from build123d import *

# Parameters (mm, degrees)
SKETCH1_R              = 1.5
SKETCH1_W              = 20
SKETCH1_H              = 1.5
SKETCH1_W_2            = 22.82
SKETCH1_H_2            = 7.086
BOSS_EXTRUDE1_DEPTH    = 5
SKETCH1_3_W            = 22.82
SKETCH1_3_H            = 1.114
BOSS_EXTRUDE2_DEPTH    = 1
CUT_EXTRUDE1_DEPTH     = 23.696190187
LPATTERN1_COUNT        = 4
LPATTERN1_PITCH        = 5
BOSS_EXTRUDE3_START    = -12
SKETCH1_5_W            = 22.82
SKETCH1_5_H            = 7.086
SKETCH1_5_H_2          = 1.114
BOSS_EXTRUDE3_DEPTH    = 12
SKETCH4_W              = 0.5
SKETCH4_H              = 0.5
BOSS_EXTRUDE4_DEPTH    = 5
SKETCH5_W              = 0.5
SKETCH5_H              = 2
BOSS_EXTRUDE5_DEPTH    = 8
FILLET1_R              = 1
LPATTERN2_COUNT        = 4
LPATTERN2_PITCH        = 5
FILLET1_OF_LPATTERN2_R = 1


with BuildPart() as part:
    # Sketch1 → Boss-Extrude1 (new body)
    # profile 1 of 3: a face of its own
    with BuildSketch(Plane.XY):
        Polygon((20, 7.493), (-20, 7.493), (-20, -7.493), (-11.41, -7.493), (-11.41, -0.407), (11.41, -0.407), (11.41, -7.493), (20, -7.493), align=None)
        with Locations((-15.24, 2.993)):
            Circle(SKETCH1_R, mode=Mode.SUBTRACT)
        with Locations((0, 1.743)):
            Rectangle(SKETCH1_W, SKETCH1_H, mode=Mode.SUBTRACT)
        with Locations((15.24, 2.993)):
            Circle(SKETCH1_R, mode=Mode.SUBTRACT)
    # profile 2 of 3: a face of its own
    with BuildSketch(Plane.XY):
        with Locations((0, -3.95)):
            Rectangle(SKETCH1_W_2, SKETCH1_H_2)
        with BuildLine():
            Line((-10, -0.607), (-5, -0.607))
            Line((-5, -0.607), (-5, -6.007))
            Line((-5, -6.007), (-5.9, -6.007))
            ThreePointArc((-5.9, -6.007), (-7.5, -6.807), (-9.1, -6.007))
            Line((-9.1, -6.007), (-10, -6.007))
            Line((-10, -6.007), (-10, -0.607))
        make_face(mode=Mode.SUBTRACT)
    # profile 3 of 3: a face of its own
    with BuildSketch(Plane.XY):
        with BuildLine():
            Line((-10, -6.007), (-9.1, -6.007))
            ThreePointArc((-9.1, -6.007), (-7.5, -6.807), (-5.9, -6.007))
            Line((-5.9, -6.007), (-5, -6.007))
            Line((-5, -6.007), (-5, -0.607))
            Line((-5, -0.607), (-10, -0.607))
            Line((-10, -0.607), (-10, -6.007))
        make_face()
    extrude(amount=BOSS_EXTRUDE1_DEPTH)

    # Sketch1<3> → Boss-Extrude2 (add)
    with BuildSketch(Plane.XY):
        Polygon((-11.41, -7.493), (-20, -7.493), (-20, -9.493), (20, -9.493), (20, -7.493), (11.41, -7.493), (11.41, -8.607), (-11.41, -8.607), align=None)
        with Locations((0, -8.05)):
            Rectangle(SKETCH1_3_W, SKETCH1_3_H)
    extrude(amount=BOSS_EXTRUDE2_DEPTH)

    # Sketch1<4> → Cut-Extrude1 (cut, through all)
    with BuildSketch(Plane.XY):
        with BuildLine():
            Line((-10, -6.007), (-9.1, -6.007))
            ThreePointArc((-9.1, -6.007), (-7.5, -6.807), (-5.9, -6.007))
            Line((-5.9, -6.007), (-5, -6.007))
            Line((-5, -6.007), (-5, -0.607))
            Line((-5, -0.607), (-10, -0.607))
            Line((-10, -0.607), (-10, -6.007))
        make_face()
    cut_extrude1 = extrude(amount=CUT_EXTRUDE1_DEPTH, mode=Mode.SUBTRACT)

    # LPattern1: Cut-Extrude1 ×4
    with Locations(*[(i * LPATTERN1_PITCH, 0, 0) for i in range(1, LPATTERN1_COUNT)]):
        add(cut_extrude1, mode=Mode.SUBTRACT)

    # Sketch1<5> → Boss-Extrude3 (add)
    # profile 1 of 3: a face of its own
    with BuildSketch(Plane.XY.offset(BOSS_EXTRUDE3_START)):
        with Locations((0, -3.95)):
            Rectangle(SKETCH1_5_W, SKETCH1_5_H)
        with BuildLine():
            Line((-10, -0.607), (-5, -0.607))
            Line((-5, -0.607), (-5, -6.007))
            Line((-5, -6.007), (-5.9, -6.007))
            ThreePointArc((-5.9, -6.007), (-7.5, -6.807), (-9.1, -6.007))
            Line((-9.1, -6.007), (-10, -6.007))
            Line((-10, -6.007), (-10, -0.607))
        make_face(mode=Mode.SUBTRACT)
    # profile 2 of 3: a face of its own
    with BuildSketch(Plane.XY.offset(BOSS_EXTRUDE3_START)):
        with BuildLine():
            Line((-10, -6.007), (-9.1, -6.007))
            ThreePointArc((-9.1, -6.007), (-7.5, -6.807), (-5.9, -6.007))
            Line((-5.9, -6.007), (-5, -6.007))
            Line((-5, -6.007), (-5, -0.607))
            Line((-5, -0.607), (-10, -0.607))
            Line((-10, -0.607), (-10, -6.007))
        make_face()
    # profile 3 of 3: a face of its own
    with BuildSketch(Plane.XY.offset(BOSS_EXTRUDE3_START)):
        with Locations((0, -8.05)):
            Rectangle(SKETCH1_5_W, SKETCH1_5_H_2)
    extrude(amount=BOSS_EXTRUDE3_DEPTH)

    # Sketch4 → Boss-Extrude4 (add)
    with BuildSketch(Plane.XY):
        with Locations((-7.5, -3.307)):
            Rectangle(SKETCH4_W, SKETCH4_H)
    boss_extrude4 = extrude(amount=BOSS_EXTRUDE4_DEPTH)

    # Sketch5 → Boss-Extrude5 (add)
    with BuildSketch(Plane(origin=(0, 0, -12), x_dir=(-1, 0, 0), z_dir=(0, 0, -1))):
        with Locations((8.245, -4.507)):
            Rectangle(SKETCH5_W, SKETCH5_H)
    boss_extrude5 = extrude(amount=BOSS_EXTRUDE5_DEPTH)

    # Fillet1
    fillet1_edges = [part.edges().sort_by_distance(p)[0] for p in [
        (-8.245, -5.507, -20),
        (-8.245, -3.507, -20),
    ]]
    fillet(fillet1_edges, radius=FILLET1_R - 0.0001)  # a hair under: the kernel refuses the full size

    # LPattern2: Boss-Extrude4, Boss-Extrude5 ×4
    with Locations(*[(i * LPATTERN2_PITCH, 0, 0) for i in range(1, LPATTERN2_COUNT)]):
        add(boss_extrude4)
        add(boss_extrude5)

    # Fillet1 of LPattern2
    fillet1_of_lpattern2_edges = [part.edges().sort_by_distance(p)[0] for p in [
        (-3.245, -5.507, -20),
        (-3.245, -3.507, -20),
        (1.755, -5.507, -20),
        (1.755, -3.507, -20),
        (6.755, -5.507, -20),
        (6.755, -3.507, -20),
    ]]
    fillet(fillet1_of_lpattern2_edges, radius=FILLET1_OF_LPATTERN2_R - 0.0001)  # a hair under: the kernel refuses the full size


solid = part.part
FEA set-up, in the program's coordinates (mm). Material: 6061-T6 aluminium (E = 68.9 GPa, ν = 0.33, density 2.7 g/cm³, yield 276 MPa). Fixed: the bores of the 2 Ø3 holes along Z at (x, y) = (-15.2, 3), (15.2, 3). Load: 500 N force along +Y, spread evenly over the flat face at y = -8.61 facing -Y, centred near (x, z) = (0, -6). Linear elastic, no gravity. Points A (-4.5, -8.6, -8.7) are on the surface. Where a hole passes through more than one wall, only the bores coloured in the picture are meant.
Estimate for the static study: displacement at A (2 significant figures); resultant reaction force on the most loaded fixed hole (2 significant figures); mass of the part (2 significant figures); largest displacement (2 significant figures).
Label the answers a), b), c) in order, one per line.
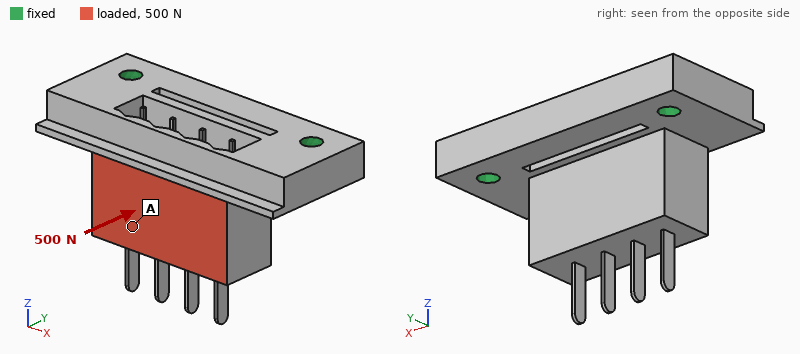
a) 44 µm
b) 270 N
c) 12 g
d) 74 µm
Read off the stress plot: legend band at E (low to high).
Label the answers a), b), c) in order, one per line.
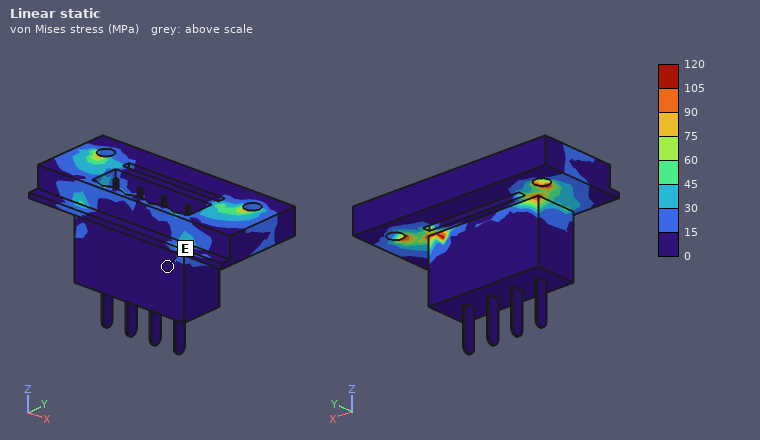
a) 0 to 15 MPa
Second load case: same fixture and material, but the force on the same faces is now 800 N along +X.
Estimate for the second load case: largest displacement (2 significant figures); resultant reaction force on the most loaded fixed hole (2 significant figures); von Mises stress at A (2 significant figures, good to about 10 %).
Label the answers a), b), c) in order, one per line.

a) 11 µm
b) 530 N
c) 9.6 MPa
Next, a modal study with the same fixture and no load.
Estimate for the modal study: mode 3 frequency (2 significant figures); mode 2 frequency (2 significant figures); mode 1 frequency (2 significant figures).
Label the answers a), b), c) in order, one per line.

a) 6600 Hz
b) 6600 Hz
c) 6600 Hz
